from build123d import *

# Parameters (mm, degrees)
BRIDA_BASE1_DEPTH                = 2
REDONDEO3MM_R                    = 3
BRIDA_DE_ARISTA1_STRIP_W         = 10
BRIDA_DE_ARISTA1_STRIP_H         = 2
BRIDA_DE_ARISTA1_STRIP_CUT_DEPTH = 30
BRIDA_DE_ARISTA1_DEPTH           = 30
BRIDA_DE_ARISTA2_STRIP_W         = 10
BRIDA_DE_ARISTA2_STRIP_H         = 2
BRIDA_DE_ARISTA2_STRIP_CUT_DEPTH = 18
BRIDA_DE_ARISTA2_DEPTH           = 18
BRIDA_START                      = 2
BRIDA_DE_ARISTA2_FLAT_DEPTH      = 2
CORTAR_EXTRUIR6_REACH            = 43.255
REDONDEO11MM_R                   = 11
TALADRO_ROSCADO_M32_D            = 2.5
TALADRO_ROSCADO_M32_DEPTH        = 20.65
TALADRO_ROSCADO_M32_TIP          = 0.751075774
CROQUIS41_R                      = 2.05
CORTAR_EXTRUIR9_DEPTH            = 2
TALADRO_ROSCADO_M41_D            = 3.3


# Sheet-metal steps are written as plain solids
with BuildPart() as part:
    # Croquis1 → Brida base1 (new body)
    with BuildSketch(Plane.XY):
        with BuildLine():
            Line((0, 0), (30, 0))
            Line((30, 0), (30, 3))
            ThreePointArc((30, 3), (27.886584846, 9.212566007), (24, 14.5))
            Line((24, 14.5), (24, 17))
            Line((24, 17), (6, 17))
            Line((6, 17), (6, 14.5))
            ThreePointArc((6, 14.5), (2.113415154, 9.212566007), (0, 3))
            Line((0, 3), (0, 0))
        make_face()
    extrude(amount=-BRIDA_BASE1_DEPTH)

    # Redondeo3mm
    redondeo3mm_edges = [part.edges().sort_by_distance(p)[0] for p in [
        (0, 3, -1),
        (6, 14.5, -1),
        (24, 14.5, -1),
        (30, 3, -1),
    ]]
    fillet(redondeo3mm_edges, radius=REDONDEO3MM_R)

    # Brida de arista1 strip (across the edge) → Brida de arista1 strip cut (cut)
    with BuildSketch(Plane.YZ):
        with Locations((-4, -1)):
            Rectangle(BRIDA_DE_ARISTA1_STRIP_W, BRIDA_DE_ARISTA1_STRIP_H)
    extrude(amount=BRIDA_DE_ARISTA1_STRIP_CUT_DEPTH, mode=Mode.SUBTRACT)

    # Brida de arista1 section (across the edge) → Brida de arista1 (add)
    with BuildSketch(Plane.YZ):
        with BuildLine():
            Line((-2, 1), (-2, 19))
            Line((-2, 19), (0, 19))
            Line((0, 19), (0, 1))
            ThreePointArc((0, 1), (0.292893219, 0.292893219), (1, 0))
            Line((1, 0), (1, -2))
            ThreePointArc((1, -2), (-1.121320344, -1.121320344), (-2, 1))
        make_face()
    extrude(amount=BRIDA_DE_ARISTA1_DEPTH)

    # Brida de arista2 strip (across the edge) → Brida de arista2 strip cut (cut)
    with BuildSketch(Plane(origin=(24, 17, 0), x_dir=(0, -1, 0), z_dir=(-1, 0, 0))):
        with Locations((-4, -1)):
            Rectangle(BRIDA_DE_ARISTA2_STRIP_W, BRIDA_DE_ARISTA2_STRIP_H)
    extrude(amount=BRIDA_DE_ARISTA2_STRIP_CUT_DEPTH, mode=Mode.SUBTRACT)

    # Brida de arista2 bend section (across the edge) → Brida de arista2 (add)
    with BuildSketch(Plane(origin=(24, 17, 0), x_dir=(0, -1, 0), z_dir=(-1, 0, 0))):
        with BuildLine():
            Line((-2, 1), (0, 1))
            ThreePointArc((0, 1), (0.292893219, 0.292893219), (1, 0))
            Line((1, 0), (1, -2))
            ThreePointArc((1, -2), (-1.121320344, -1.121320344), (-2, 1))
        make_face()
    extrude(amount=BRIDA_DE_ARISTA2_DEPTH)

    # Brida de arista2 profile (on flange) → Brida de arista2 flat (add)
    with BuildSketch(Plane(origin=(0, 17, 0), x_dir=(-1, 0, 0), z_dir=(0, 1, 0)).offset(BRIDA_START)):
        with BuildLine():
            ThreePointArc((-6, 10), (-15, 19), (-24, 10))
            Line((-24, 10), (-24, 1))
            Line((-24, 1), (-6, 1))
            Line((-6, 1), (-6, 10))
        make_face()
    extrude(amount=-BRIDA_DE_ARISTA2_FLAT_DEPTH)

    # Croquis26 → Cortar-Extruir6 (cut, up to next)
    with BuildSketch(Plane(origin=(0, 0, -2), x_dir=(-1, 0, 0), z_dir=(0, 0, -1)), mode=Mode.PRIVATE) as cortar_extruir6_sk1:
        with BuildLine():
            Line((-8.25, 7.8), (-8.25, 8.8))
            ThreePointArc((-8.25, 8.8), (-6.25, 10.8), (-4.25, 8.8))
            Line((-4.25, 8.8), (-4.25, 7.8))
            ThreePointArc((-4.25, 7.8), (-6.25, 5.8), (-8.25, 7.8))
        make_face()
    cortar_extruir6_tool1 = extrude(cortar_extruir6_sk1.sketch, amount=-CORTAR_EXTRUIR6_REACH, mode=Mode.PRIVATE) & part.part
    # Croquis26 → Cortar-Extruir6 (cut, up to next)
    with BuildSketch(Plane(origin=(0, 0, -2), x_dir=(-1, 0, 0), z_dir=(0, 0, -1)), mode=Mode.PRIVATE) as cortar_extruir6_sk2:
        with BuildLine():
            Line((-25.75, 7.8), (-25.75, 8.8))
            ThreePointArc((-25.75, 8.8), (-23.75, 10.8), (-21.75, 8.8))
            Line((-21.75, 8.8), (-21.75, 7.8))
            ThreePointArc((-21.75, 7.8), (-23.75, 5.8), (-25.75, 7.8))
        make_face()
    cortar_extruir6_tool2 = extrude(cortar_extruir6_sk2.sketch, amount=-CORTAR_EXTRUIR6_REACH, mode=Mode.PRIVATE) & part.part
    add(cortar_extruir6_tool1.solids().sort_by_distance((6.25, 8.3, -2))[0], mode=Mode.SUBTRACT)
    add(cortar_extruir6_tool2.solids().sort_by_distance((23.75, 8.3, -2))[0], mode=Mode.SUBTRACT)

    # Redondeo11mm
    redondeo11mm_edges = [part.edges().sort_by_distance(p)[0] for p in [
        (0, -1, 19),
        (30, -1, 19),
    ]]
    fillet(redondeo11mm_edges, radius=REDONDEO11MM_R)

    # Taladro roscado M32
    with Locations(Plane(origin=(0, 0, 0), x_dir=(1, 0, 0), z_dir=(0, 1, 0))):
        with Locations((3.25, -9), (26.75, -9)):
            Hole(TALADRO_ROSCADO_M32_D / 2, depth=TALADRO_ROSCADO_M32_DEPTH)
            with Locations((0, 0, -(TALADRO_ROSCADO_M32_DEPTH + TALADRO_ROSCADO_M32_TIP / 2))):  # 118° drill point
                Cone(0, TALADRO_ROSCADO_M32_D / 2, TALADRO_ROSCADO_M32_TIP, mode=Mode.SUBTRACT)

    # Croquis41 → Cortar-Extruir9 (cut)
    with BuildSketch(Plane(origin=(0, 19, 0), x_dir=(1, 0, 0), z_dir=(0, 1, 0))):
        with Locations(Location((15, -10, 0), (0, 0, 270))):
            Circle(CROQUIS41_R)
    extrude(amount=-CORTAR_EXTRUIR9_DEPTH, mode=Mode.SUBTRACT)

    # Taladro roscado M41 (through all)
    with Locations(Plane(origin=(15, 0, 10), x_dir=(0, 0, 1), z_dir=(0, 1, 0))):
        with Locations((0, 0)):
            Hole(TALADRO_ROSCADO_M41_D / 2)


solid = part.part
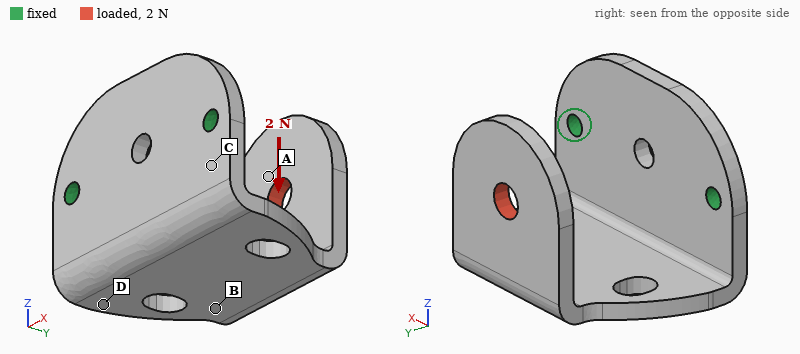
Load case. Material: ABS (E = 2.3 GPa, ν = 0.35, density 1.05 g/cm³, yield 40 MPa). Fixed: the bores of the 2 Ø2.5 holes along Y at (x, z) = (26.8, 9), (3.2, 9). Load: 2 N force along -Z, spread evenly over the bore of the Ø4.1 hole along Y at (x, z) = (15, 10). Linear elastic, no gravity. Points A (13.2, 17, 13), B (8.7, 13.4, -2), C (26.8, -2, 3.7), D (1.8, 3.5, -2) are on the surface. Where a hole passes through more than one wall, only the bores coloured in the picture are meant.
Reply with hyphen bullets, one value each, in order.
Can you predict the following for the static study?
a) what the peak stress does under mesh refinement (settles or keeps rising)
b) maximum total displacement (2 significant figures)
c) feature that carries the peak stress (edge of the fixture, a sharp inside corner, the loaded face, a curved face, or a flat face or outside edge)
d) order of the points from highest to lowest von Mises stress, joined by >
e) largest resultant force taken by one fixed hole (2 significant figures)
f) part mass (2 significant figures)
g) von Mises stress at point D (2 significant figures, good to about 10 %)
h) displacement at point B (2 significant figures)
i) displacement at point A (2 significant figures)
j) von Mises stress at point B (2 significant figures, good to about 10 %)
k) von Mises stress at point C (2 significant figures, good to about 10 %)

- keeps rising
- 0.41 mm
- edge of the fixture
- C > D > B > A
- 1.1 N
- 2.6 g
- 1.4 MPa
- 0.19 mm
- 0.31 mm
- 0.77 MPa
- 1.9 MPa
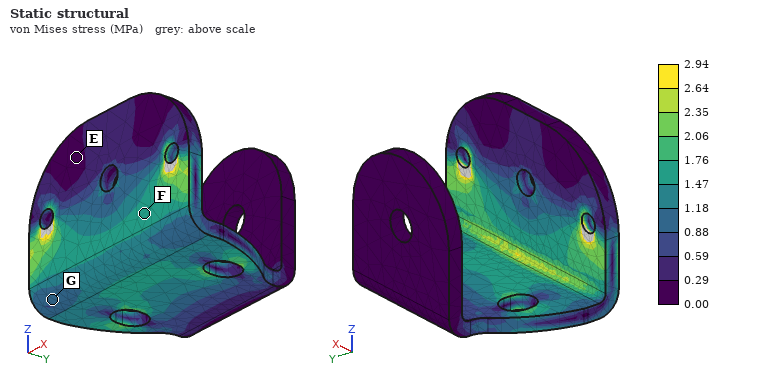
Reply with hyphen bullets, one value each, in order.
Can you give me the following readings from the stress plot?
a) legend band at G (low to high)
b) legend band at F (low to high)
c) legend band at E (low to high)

- 0.88 to 1.18 MPa
- 1.47 to 1.76 MPa
- 0.00 to 0.29 MPa
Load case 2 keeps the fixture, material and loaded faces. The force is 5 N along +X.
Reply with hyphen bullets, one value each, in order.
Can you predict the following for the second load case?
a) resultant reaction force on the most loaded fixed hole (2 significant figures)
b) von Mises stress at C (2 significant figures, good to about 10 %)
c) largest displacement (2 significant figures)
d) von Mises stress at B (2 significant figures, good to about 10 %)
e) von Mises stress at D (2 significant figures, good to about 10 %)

- 4.8 N
- 2.7 MPa
- 0.49 mm
- 3.1 MPa
- 1.5 MPa
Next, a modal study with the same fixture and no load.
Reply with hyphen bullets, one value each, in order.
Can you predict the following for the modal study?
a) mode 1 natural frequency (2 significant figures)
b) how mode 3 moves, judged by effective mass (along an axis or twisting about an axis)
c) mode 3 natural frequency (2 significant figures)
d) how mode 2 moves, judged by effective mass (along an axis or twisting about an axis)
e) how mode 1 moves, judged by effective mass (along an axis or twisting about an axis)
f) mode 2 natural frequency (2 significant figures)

- 420 Hz
- along Y
- 960 Hz
- along X
- along Z
- 750 Hz
